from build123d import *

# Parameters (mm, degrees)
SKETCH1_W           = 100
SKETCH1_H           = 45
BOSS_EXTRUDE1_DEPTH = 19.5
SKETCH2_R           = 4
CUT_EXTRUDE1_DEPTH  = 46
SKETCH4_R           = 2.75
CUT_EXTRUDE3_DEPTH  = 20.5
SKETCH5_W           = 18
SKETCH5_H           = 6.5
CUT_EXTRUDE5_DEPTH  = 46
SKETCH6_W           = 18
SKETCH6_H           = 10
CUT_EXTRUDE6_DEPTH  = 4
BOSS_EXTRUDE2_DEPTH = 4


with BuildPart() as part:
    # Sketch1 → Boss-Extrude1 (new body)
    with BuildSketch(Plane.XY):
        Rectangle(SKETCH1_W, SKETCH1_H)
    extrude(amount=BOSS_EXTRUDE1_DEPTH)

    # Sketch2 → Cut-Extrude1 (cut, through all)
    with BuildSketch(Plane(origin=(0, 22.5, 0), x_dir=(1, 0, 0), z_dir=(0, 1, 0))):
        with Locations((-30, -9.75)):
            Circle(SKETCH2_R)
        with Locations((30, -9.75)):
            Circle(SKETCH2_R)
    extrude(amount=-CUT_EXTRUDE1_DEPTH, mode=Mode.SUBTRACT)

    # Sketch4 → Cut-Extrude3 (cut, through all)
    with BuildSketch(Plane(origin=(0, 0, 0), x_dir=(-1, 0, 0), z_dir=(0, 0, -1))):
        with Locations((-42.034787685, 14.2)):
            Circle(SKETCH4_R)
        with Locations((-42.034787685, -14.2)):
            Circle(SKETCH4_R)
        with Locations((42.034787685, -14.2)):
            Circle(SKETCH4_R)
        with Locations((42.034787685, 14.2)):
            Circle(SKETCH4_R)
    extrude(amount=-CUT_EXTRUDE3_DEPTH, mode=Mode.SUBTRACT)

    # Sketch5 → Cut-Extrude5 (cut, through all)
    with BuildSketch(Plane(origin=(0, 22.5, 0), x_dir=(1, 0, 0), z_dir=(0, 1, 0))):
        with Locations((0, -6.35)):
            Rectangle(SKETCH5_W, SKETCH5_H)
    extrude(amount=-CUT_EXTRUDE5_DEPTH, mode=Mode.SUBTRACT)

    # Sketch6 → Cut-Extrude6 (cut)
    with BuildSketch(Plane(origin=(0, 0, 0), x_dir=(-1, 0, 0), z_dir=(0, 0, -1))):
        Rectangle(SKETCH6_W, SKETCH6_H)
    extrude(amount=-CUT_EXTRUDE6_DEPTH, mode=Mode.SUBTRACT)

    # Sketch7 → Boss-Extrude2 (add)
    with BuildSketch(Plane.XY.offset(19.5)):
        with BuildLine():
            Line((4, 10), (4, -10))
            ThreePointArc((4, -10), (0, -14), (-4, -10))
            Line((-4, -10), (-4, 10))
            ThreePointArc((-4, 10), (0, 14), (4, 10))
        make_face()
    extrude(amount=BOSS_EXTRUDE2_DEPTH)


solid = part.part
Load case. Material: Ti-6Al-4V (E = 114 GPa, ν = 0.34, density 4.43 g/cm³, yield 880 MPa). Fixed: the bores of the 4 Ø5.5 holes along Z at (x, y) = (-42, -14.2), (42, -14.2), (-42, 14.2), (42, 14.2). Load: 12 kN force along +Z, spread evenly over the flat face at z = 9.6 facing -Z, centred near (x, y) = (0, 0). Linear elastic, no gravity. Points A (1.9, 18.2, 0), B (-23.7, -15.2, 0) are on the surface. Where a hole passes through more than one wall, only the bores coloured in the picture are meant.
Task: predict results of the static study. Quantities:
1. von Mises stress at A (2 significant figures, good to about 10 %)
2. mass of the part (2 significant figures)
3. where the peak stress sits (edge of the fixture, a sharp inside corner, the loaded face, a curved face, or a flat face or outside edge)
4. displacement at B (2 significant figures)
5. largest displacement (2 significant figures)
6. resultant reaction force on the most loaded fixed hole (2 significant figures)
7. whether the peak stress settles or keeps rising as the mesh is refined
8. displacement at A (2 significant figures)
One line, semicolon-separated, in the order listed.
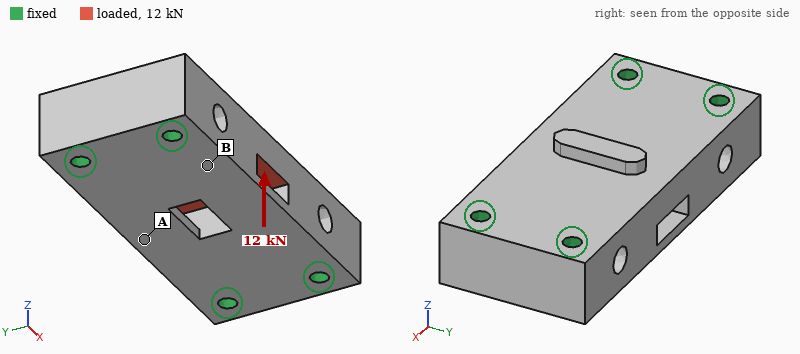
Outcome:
38 MPa; 340 g; edge of the fixture; 15 µm; 29 µm; 3.1 kN; keeps rising; 22 µm
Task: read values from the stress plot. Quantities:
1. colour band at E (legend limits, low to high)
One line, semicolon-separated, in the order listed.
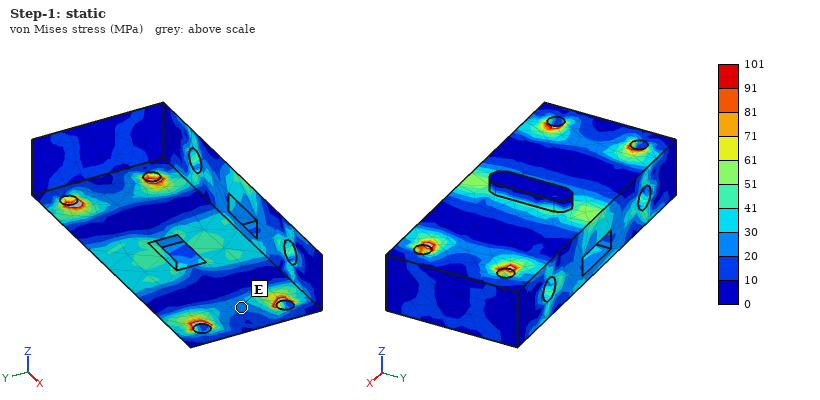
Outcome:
20 to 30 MPa
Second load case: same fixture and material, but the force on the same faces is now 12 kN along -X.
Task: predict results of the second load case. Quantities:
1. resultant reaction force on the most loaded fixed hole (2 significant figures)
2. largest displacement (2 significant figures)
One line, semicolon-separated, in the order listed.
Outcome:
3.0 kN; 6.0 µm
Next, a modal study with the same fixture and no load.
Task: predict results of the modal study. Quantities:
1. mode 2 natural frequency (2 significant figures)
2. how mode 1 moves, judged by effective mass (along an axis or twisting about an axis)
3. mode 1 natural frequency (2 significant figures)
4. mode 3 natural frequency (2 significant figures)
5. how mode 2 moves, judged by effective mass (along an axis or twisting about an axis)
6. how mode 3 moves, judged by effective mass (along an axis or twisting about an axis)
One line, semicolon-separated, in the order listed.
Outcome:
14 kHz; along Z; 9700 Hz; 15 kHz; along Y; along Y
